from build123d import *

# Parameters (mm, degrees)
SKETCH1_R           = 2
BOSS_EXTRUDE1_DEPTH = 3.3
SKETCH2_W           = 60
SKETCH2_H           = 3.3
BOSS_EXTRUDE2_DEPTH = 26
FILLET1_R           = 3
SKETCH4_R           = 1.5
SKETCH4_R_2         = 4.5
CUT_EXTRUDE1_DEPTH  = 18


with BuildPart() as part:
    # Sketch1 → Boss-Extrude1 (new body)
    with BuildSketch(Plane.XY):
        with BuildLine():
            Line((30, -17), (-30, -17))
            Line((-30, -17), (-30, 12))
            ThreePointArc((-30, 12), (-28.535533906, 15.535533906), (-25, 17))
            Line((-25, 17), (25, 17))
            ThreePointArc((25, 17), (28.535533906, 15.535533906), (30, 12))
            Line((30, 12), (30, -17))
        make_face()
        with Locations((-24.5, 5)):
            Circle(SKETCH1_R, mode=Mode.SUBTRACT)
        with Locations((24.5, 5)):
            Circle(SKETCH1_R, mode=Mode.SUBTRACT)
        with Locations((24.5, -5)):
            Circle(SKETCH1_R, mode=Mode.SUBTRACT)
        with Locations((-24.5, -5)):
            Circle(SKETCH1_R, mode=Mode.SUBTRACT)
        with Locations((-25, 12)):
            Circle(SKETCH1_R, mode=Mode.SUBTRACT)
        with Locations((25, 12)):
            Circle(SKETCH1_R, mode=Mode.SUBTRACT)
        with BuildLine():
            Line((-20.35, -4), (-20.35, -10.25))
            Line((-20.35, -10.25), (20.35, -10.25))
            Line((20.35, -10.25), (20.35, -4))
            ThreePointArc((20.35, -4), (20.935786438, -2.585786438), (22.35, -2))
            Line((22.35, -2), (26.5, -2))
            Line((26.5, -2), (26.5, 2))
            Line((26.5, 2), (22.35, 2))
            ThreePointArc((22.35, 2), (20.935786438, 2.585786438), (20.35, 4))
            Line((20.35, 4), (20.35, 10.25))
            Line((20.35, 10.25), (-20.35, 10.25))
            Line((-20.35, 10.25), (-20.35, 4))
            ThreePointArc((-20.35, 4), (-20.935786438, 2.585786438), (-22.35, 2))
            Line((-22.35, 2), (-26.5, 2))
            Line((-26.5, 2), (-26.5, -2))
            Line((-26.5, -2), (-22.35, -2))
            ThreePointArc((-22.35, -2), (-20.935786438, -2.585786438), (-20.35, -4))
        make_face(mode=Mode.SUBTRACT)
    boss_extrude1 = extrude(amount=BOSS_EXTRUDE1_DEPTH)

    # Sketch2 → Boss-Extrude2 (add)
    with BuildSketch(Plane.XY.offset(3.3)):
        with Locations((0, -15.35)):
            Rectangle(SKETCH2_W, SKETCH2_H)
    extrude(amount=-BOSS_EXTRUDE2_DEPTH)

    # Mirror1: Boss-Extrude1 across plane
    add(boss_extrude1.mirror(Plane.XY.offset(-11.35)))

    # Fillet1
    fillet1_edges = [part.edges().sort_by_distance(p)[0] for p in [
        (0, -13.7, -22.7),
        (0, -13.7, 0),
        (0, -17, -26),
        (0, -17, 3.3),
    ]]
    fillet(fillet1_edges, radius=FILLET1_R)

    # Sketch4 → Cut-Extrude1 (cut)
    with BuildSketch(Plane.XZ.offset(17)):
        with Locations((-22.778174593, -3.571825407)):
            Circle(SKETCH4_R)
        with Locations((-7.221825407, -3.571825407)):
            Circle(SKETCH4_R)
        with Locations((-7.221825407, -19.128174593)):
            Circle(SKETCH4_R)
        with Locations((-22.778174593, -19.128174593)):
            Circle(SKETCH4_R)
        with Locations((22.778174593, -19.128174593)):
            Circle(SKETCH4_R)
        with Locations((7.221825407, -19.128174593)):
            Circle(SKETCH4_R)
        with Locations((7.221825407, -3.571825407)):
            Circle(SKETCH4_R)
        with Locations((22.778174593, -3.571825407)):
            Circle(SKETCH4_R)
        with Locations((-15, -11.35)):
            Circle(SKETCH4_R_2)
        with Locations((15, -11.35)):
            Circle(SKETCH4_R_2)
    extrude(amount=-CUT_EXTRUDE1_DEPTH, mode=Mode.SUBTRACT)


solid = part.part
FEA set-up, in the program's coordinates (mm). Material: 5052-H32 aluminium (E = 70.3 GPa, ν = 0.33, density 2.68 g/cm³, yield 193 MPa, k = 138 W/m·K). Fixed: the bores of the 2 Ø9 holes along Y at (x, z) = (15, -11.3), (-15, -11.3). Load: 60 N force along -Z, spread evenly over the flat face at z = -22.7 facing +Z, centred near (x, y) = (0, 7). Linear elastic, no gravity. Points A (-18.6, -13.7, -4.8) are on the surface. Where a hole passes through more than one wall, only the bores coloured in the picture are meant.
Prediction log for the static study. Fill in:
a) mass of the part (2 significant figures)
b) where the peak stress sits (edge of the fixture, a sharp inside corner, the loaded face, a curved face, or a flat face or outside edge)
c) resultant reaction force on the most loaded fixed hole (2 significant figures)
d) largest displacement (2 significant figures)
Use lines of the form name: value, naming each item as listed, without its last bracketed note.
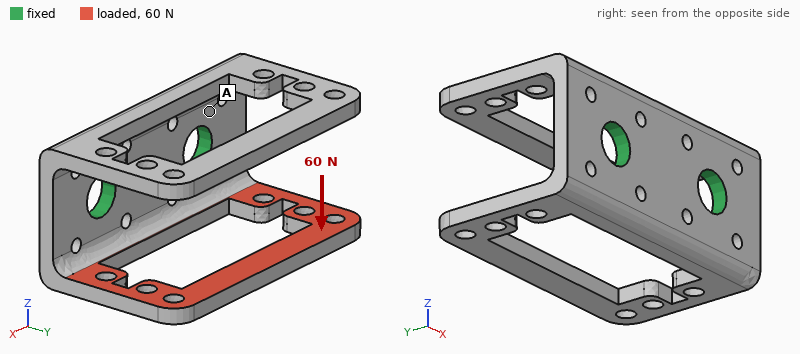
mass of the part: 29 g
where the peak stress sits: a curved face
resultant reaction force on the most loaded fixed hole: 30 N
largest displacement: 0.21 mm
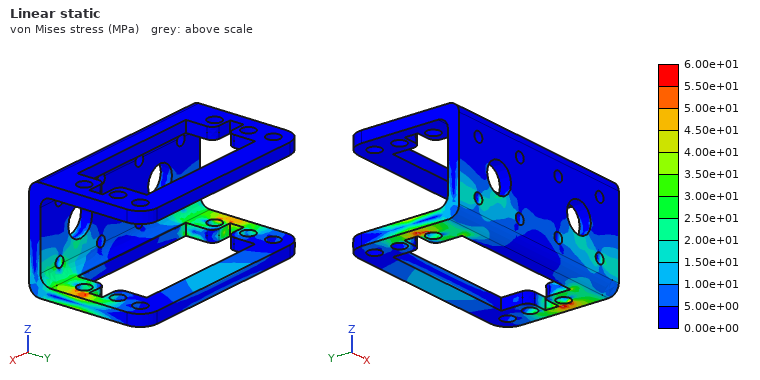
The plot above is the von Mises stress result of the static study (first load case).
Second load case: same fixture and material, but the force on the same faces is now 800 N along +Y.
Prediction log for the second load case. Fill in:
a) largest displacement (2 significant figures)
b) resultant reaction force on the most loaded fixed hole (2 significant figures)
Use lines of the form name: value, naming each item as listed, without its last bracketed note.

largest displacement: 0.21 mm
resultant reaction force on the most loaded fixed hole: 440 N
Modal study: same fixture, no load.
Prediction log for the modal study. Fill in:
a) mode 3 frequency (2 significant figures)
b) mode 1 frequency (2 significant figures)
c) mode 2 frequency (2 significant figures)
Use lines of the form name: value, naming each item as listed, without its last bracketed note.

mode 3 frequency: 2700 Hz
mode 1 frequency: 1300 Hz
mode 2 frequency: 1300 Hz
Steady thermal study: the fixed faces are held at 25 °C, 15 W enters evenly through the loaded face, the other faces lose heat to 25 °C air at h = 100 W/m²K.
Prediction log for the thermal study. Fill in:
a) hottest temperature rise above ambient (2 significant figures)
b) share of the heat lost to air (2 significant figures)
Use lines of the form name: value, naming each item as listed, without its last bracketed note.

hottest temperature rise above ambient: 49 K
share of the heat lost to air: 43 %
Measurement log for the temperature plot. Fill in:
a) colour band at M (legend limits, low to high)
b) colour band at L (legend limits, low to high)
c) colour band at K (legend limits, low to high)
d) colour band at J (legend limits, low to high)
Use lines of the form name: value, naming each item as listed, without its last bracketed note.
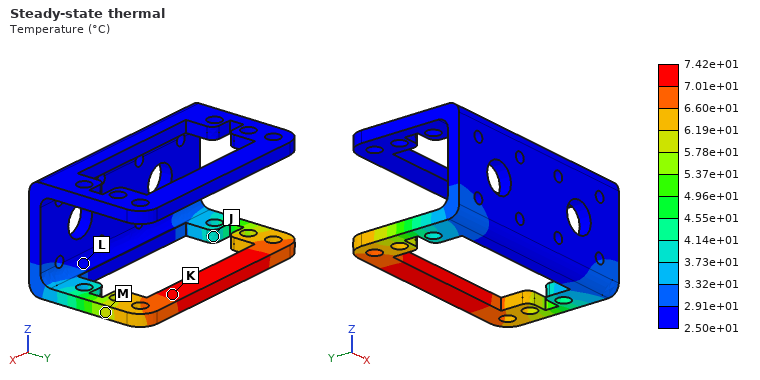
colour band at M: 5.78e+01 to 6.19e+01 °C
colour band at L: 2.50e+01 to 2.91e+01 °C
colour band at K: 7.01e+01 to 7.42e+01 °C
colour band at J: 3.73e+01 to 4.14e+01 °C
